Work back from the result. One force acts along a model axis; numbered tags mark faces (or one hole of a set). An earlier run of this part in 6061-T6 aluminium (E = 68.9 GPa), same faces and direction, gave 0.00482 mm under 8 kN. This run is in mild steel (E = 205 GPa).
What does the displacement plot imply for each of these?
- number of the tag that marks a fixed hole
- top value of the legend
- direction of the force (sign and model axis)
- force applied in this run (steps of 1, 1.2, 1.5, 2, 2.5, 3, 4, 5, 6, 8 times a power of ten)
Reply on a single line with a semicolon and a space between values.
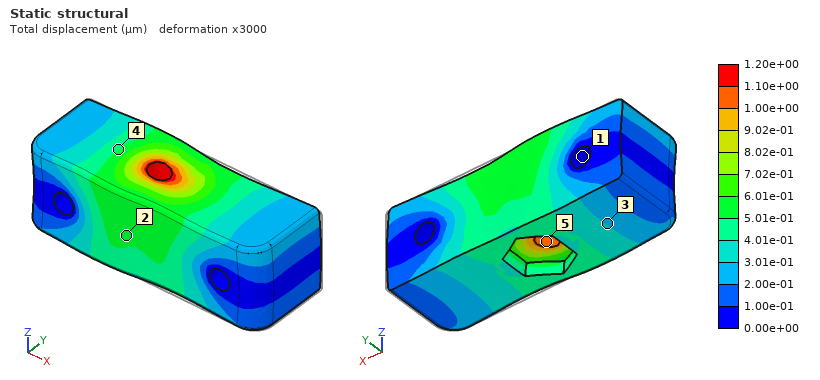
1; 1.20e+00 µm; -X; 6 kN
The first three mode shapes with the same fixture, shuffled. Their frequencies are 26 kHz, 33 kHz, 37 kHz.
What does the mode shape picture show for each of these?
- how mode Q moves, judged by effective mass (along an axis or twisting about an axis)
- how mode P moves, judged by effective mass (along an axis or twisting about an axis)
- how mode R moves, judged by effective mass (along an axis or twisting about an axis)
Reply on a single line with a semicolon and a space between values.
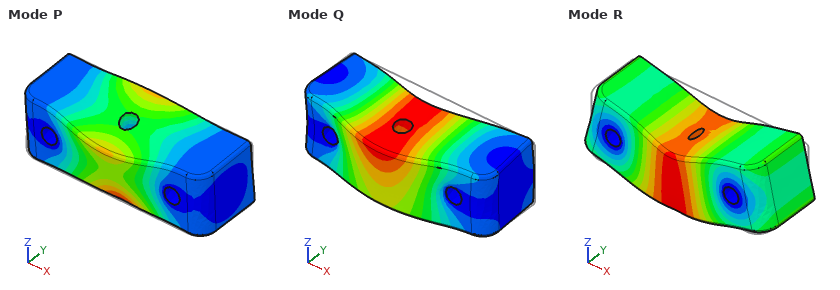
along Y; twisting about X; along Z
